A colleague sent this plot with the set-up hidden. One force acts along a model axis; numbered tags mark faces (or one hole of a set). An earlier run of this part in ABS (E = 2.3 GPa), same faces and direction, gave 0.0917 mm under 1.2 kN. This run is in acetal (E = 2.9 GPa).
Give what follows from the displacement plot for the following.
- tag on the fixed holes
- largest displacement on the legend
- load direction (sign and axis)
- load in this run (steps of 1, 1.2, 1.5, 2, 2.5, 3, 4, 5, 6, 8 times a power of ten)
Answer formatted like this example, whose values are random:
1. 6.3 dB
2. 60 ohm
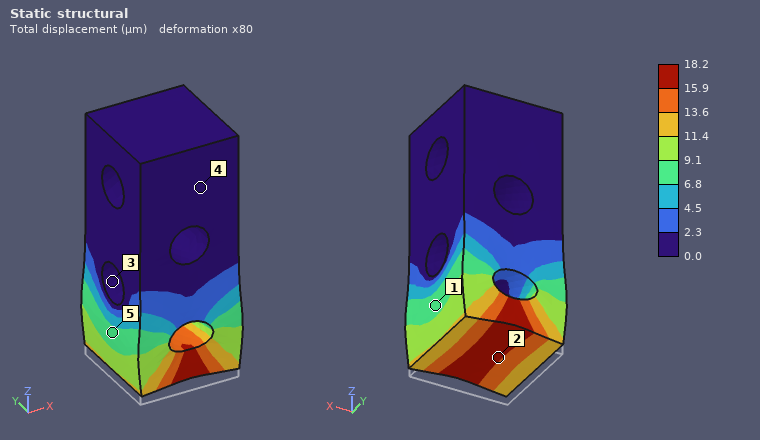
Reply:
1. 3
2. 18.2 µm
3. +Z
4. 300 N
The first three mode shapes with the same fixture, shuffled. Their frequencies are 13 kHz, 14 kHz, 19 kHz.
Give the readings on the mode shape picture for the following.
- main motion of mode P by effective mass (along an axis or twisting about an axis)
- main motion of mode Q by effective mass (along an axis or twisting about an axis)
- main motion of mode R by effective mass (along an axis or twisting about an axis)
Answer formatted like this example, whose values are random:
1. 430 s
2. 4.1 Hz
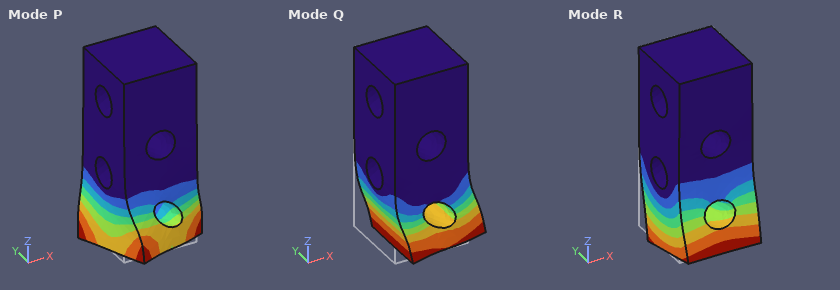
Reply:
1. twisting about Z
2. along X
3. along Y
